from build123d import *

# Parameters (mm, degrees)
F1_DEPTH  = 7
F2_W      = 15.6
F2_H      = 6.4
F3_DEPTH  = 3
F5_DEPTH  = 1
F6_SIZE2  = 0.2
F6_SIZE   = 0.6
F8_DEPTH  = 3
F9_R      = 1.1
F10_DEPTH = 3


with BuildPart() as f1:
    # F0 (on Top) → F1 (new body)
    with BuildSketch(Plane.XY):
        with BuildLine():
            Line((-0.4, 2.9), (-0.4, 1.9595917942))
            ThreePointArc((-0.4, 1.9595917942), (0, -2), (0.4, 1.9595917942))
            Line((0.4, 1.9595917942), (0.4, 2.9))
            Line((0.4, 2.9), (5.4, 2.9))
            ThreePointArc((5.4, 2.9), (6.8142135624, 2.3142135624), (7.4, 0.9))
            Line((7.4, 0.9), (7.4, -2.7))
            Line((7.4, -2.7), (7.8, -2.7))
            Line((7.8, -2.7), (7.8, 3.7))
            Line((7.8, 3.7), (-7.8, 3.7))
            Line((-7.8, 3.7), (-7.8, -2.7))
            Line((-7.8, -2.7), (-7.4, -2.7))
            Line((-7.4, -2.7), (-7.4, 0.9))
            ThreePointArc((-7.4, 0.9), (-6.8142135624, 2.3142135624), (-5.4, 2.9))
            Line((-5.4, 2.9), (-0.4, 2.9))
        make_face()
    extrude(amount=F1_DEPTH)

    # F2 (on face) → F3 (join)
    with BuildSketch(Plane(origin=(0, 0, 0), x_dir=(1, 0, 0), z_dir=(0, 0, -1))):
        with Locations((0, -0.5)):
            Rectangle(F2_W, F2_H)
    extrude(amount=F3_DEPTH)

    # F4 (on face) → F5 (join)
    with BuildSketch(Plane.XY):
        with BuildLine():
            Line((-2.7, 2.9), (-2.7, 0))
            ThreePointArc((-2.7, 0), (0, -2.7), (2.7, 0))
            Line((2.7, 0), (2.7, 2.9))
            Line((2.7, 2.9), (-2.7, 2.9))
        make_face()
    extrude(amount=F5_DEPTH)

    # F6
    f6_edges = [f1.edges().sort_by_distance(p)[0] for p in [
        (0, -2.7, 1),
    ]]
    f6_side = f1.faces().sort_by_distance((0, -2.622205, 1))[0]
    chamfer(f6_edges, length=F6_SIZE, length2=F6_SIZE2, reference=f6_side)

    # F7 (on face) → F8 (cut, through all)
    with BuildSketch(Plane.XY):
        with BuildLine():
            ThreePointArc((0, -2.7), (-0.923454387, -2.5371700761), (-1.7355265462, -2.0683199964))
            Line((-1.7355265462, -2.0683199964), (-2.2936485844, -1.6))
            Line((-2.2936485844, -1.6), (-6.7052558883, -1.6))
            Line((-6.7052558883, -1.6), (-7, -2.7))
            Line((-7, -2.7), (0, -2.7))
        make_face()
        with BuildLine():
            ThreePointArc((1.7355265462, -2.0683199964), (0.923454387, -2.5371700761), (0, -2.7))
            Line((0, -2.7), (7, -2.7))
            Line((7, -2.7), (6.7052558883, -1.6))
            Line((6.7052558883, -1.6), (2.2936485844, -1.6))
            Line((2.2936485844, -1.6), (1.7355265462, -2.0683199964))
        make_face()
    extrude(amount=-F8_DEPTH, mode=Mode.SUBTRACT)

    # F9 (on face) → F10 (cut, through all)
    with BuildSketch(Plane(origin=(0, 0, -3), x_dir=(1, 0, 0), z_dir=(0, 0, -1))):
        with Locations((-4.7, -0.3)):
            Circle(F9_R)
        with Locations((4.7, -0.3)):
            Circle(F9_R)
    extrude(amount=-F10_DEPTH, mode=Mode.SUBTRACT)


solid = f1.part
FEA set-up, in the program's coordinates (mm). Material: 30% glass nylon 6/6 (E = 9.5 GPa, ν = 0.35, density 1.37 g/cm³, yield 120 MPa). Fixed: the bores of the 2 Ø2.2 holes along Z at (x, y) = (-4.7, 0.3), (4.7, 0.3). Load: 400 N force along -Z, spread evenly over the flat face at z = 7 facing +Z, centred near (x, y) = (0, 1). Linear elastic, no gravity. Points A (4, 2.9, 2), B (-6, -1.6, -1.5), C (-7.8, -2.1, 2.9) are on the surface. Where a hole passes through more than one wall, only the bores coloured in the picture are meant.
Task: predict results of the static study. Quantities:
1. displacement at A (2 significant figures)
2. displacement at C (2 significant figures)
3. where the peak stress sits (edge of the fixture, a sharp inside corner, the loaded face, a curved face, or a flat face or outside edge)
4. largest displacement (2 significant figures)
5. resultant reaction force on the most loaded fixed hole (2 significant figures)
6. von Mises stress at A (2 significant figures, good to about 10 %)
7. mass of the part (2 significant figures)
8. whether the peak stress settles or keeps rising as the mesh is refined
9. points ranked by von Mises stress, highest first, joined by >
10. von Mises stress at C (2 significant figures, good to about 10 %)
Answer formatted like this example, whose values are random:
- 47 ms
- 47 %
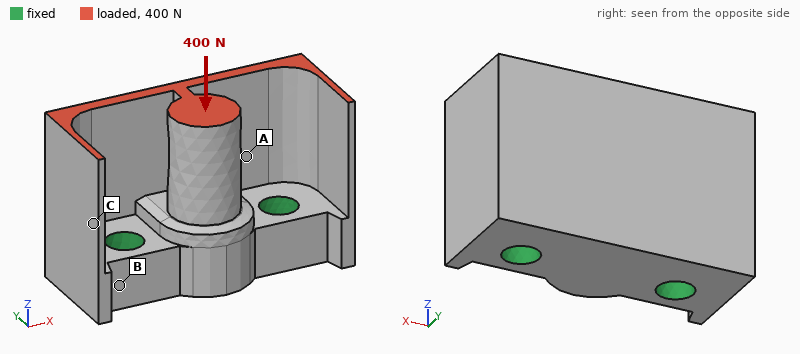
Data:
- 13 µm
- 9.0 µm
- edge of the fixture
- 24 µm
- 200 N
- 15 MPa
- 0.66 g
- keeps rising
- A > C > B
- 11 MPa
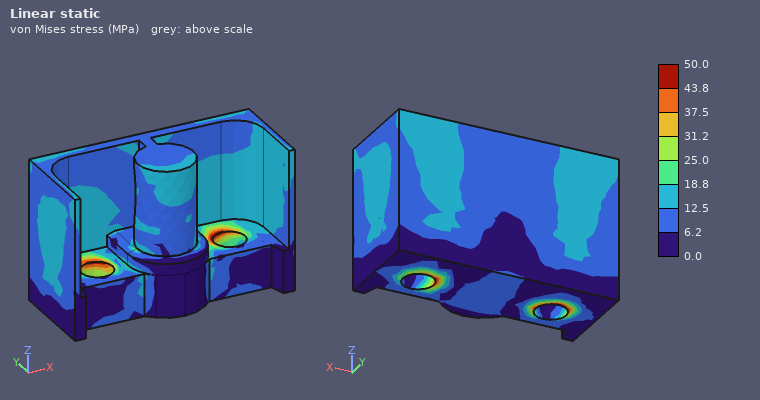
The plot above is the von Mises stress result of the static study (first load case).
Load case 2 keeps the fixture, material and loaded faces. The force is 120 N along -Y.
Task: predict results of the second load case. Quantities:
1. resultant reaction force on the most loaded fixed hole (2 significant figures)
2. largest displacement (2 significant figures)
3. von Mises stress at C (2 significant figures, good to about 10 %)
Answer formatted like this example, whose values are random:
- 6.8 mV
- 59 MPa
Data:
- 61 N
- 0.12 mm
- 20 MPa
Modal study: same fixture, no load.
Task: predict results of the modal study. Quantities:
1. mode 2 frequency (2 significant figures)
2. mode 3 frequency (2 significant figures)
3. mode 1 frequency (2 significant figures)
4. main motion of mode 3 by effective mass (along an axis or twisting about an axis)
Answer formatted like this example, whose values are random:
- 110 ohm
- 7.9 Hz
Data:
- 11 kHz
- 17 kHz
- 11 kHz
- along Y
